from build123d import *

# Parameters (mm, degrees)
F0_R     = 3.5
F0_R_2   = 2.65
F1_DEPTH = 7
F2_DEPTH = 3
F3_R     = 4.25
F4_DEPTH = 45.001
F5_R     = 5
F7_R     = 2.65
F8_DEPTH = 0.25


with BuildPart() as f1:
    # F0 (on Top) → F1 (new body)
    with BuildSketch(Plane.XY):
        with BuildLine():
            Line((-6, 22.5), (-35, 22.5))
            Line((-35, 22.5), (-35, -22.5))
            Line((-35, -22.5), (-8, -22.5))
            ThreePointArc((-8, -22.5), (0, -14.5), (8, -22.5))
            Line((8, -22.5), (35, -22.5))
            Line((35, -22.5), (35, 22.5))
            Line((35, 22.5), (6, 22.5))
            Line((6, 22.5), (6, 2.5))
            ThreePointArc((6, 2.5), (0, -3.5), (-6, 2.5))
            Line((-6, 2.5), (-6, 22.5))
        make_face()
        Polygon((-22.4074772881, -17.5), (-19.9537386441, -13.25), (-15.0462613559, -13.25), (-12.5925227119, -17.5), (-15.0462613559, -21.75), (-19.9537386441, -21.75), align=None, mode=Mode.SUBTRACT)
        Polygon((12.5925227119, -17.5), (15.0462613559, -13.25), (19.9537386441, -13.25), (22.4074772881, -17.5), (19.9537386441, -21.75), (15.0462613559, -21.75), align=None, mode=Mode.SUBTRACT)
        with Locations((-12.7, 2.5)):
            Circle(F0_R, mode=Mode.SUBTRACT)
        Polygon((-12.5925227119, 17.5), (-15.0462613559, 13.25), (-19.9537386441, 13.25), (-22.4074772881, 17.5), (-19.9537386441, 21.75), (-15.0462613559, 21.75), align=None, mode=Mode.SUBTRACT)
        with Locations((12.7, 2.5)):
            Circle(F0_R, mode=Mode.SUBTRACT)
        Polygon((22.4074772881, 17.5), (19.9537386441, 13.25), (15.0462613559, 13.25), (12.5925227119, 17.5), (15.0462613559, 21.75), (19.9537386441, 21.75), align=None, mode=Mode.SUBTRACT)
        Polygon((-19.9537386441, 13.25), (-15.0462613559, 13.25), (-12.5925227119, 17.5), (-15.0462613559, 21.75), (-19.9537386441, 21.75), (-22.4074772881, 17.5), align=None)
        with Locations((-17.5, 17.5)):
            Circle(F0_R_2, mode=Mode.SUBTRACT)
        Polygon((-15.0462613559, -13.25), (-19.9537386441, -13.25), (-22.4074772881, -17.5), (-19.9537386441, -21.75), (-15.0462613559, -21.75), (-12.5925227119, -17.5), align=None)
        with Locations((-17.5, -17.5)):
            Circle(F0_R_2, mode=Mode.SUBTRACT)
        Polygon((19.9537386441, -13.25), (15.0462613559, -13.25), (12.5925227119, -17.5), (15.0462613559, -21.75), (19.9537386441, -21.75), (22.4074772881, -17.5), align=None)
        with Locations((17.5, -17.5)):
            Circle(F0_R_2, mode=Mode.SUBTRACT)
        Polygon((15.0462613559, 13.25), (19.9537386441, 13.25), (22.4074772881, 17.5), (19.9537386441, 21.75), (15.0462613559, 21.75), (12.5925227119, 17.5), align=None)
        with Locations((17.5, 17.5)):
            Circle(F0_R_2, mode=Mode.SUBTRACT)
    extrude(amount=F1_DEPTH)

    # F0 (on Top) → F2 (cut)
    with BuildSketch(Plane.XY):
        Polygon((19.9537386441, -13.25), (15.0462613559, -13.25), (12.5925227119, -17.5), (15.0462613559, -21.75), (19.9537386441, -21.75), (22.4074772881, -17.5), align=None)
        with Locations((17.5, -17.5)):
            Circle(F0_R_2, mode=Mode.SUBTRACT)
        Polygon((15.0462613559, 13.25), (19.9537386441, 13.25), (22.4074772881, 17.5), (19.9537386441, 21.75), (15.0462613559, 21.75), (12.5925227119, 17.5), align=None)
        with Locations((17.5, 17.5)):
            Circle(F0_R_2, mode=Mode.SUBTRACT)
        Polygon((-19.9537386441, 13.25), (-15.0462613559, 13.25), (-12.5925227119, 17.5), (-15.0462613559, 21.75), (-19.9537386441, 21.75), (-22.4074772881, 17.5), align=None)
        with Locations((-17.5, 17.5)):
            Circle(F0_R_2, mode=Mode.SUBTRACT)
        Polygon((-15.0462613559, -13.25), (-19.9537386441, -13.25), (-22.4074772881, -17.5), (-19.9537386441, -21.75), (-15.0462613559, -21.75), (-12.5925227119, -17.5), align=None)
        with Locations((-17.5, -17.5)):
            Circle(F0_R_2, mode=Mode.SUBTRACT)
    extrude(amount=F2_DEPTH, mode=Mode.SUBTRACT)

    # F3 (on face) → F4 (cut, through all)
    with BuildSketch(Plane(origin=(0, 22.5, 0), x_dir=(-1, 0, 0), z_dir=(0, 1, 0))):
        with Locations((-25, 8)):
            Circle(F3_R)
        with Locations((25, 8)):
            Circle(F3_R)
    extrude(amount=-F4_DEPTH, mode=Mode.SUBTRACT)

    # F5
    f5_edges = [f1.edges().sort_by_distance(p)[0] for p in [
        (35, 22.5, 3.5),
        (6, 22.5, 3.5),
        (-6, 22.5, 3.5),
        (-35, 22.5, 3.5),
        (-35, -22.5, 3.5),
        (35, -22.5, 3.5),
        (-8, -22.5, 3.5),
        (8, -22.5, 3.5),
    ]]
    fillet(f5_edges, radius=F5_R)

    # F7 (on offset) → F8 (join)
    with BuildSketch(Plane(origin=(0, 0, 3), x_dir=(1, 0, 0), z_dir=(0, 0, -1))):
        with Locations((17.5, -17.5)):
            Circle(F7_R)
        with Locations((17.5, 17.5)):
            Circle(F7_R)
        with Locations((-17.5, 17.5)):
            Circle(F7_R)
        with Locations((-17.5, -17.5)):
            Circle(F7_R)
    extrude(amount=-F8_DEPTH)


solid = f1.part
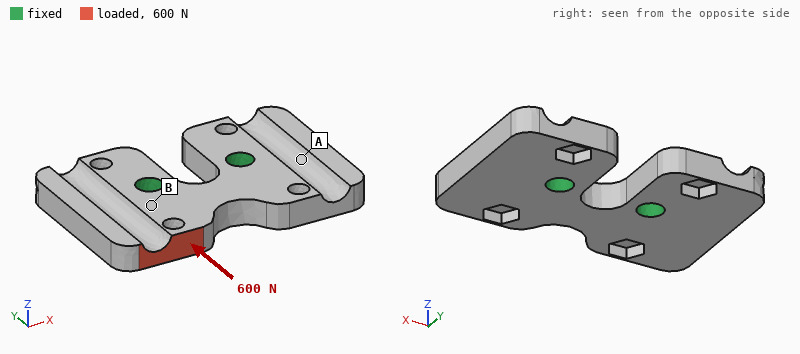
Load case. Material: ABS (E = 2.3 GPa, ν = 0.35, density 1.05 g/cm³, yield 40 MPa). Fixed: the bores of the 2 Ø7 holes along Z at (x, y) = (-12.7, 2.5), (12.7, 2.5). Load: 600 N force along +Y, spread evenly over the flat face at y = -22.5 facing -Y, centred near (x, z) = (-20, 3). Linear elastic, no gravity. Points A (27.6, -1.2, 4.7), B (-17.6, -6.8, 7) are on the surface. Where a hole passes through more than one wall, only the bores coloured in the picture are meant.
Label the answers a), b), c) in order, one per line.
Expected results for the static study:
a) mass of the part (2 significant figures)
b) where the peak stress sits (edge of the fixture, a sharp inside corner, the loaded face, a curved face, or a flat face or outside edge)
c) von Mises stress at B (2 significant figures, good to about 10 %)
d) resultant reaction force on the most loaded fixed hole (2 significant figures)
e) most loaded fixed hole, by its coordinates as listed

a) 16 g
b) a flat face or outside edge
c) 5.5 MPa
d) 660 N
e) (-12.7, 2.5)
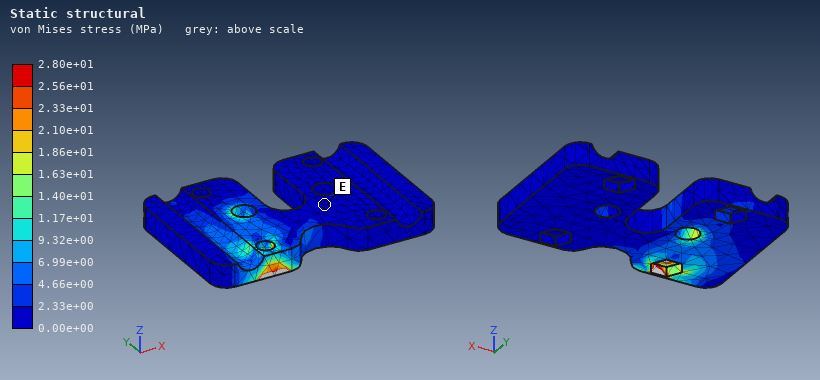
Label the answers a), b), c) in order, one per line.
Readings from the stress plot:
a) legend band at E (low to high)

a) 0.00e+00 to 2.33e+00 MPa
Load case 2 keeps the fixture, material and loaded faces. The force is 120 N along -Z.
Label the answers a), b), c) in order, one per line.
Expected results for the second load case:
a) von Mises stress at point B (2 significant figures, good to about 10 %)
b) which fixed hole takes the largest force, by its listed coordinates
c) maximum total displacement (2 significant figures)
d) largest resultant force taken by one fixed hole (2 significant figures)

a) 8.8 MPa
b) (-12.7, 2.5)
c) 0.47 mm
d) 130 N
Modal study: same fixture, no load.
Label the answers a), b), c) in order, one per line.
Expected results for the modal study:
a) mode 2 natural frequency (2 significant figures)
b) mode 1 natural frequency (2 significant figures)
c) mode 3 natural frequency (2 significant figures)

a) 2300 Hz
b) 2200 Hz
c) 2500 Hz
